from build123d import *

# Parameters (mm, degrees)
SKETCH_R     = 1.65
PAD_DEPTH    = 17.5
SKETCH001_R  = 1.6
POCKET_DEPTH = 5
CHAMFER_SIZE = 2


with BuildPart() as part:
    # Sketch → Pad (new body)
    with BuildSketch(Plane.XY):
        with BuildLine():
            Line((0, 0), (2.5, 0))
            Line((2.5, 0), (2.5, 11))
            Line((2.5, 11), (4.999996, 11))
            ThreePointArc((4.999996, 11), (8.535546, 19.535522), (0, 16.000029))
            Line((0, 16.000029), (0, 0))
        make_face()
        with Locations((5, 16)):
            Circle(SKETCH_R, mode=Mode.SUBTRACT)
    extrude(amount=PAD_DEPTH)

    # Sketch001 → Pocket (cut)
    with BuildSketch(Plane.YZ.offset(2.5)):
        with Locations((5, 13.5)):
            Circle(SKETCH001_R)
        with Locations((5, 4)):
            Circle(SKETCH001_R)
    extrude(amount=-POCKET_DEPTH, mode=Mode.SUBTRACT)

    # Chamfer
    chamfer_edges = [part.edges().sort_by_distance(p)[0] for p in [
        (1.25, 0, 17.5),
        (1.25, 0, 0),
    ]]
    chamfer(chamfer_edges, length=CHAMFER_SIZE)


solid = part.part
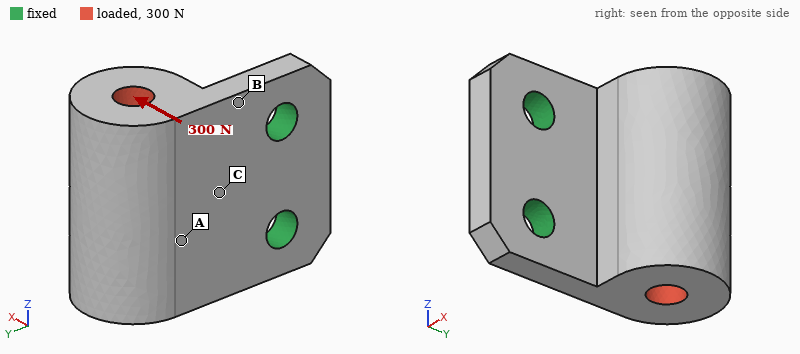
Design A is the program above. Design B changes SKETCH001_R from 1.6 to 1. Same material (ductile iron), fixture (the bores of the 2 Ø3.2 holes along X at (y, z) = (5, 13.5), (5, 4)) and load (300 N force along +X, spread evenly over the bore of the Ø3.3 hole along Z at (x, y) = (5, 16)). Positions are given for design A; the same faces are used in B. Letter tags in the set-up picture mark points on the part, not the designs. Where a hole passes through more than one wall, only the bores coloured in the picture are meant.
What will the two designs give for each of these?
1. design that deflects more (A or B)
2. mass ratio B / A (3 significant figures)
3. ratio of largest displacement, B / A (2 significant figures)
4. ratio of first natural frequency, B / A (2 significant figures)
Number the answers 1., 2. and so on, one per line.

1. B
2. 1.01
3. 1.2
4. 0.90
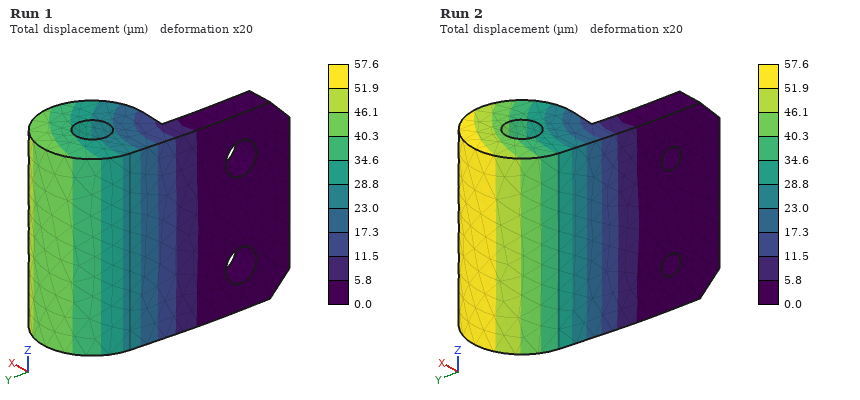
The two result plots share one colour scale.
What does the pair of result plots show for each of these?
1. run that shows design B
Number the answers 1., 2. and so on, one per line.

1. Run 2
